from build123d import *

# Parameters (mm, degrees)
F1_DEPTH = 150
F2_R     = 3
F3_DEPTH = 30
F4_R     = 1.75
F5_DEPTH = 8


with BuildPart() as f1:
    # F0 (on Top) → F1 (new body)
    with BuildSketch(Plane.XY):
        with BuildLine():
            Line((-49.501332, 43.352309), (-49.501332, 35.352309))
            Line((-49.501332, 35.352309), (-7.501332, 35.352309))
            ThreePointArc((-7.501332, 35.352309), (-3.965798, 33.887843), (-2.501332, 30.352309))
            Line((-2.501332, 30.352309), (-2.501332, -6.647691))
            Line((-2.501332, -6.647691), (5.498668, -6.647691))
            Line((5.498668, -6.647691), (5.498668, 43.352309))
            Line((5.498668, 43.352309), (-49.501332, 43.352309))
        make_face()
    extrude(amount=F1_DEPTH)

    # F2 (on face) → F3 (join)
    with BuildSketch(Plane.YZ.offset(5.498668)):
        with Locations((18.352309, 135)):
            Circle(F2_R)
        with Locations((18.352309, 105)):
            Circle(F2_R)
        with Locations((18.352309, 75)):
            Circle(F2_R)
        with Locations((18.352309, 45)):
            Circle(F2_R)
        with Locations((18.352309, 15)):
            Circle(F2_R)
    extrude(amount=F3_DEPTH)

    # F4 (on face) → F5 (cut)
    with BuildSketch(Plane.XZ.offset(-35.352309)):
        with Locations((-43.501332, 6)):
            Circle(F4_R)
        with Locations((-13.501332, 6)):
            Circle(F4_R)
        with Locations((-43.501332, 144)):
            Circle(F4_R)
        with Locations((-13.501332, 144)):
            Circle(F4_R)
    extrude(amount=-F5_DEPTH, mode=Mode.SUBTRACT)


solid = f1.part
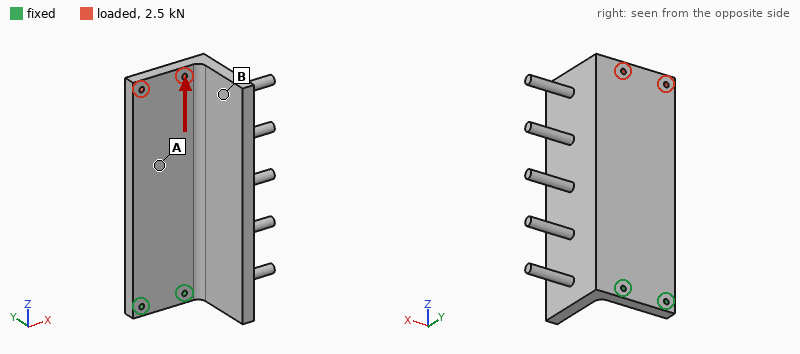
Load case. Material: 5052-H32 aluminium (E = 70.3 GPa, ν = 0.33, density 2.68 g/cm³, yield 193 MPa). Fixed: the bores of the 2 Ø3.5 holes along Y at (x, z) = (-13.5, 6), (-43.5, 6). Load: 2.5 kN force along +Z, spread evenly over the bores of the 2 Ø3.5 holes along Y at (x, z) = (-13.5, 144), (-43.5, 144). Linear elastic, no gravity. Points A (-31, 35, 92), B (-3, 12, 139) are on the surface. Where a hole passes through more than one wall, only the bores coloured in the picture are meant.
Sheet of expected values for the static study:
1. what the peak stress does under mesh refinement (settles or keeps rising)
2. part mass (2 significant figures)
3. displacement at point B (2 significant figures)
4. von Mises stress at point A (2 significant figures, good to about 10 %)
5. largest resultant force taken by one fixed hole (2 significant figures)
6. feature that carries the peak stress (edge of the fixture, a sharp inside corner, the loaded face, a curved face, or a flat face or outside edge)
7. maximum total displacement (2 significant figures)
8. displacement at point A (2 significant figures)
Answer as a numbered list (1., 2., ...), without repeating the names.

1. keeps rising
2. 320 g
3. 17 µm
4. 6.8 MPa
5. 1.3 kN
6. edge of the fixture
7. 30 µm
8. 11 µm
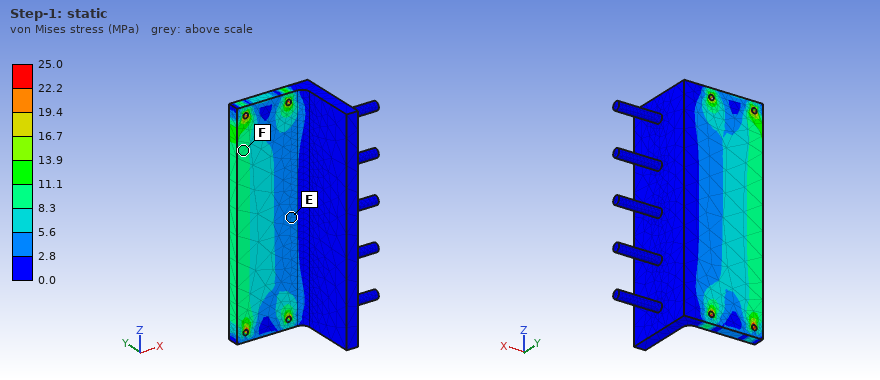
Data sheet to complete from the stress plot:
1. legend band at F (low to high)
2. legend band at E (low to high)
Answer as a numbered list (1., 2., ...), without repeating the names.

1. 8.3 to 11.1 MPa
2. 2.8 to 5.6 MPa
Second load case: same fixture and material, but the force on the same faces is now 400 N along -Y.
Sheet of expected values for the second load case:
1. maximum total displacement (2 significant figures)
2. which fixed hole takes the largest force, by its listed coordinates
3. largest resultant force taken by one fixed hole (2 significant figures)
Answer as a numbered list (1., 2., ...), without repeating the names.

1. 0.99 mm
2. (-13.5, 6)
3. 330 N
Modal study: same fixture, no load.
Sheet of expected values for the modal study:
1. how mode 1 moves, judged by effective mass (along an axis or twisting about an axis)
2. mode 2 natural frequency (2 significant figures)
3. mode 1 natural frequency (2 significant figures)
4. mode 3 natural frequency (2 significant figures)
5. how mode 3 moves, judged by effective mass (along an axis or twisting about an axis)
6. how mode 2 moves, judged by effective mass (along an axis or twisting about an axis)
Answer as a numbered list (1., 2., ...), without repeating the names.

1. along Y
2. 850 Hz
3. 310 Hz
4. 1400 Hz
5. along X
6. along X
